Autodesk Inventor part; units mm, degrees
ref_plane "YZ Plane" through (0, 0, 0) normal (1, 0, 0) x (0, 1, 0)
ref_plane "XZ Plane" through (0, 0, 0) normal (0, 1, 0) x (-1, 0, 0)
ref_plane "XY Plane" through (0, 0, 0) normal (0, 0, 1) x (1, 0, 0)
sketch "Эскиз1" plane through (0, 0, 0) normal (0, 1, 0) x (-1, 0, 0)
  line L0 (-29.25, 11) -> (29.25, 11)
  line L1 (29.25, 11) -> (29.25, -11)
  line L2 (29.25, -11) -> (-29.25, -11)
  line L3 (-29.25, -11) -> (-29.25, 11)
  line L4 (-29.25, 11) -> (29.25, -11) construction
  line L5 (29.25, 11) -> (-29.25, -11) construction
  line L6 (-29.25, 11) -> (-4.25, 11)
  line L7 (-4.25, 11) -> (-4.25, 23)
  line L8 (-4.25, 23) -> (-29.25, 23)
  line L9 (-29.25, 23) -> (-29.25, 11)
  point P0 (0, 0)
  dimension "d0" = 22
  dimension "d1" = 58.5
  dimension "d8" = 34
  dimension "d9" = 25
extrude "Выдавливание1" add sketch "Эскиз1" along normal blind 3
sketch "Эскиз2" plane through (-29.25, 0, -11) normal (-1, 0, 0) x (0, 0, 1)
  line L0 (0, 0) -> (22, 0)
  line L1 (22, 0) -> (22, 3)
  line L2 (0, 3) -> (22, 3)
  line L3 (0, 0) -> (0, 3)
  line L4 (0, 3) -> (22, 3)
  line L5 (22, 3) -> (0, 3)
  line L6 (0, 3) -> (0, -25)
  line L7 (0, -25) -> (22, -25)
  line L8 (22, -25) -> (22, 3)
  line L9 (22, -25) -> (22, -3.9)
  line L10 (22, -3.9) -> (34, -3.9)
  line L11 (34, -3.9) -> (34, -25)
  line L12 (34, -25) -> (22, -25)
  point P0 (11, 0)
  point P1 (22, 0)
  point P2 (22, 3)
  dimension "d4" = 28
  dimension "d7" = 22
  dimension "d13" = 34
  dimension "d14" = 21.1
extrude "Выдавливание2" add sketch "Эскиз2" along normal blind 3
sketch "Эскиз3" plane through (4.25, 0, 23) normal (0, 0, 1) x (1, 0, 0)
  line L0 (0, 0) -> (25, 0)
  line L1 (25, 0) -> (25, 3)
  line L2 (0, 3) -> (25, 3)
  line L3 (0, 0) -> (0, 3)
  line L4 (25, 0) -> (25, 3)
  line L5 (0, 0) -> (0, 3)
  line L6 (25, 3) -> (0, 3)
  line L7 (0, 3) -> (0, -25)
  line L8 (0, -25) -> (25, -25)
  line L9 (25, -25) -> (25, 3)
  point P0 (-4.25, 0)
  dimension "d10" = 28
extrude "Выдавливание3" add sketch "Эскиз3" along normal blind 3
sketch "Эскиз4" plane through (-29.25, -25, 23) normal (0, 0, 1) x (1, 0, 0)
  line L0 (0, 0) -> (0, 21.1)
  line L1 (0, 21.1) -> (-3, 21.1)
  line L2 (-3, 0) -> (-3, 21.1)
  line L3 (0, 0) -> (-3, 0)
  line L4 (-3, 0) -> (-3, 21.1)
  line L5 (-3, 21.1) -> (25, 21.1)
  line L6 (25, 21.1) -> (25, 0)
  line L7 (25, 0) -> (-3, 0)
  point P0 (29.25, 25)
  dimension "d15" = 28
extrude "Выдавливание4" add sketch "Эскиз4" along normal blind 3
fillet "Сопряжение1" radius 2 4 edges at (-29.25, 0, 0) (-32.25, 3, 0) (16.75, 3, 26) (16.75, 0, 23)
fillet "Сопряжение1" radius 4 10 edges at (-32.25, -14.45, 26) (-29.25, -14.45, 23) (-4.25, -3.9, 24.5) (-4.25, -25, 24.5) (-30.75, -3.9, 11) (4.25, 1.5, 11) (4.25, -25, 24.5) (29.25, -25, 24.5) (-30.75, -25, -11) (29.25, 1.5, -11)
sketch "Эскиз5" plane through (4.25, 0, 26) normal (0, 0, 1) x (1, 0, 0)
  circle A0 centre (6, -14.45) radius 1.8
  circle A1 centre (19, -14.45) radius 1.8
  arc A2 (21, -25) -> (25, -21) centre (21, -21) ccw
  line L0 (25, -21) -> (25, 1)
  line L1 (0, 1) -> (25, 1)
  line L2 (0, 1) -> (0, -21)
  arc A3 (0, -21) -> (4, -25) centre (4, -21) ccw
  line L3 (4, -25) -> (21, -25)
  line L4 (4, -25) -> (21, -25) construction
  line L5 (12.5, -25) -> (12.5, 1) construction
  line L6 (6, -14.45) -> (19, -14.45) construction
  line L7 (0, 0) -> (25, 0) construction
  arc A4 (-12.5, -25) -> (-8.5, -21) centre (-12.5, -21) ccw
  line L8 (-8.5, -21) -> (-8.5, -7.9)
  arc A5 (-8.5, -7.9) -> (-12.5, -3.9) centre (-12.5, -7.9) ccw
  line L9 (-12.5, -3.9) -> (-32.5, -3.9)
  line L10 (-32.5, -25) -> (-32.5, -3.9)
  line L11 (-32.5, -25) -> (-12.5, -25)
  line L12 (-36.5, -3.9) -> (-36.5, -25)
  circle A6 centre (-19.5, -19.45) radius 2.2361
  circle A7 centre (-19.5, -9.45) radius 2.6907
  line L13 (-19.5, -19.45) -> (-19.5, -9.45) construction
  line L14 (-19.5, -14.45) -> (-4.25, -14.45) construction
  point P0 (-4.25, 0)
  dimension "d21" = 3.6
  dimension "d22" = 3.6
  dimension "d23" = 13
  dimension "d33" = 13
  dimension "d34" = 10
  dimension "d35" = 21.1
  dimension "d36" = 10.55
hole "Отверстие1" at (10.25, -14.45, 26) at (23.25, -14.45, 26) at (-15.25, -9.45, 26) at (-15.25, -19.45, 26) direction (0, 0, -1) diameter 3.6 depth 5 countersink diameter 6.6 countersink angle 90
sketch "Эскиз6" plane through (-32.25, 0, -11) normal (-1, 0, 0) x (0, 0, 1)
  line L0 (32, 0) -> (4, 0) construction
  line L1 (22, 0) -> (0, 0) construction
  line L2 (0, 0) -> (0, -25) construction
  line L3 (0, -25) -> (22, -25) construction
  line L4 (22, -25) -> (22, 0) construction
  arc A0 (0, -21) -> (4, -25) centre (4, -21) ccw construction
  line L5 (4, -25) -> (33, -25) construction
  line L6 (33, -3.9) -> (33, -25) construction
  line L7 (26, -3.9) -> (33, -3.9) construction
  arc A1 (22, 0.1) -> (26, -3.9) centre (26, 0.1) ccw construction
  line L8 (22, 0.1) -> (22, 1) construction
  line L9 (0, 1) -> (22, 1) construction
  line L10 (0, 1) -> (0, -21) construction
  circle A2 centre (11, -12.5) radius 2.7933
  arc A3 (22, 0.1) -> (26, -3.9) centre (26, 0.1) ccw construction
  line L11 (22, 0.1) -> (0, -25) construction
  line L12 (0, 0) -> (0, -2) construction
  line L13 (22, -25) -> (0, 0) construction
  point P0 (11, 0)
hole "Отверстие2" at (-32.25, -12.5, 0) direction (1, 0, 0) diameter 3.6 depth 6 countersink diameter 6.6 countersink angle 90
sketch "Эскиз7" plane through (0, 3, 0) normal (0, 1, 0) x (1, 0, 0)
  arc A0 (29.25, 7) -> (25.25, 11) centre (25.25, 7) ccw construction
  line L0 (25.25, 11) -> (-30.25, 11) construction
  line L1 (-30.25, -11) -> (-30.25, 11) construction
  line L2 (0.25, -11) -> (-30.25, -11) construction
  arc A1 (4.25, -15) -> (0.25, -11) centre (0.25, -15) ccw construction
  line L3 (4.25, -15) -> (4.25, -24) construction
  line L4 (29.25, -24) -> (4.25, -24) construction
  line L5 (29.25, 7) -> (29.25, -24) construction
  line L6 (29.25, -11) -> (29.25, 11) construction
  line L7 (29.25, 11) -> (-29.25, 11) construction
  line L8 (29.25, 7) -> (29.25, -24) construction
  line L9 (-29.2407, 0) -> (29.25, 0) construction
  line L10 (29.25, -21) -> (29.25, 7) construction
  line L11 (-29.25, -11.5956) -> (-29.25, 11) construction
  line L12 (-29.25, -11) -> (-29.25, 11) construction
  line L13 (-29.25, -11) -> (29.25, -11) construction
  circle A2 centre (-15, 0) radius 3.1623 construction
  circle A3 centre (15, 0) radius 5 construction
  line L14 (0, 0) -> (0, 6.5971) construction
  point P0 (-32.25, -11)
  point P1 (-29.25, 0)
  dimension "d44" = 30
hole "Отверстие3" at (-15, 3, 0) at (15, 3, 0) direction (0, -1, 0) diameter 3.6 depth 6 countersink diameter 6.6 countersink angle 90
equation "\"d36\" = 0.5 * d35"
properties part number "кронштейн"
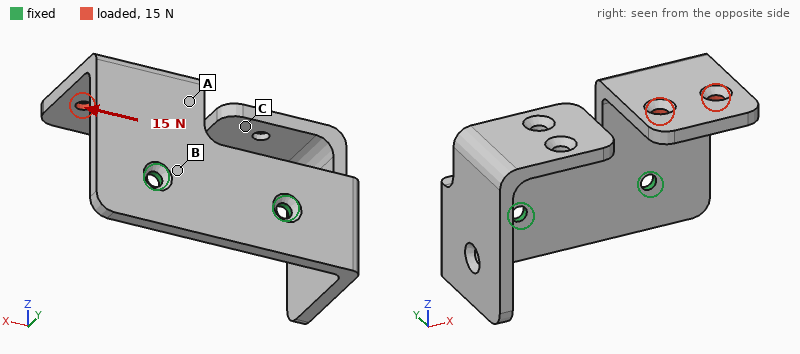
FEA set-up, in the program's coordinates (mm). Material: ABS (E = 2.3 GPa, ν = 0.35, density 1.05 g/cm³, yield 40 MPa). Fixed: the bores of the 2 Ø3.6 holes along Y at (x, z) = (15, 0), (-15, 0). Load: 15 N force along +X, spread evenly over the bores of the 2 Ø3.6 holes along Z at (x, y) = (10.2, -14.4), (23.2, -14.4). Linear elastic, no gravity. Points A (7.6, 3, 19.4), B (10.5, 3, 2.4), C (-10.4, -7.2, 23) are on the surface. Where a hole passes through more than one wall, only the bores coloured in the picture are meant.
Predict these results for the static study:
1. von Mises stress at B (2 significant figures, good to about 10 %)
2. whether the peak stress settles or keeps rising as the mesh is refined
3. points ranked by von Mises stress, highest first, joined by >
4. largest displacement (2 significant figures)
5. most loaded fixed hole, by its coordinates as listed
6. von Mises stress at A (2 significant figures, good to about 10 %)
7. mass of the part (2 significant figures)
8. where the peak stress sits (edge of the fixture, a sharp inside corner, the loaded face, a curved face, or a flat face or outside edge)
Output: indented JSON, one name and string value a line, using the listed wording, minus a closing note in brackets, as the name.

{
  "von Mises stress at B": "2.1 MPa",
  "whether the peak stress settles or keeps rising as the mesh is refined": "keeps rising",
  "points ranked by von Mises stress, highest first, joined by >": "A > B > C",
  "largest displacement": "0.76 mm",
  "most loaded fixed hole, by its coordinates as listed": "(15, 0)",
  "von Mises stress at A": "4.8 MPa",
  "mass of the part": "11 g",
  "where the peak stress sits": "edge of the fixture"
}
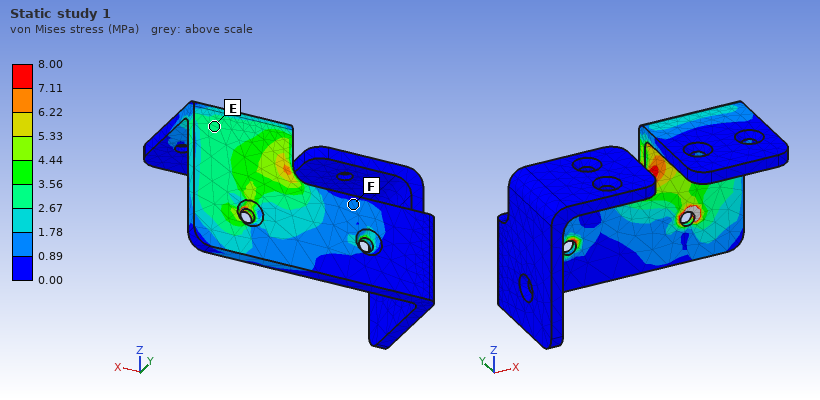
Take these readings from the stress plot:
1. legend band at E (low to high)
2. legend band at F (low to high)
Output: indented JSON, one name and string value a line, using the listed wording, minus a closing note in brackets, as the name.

{
  "legend band at E": "2.67 to 3.56 MPa",
  "legend band at F": "0.89 to 1.78 MPa"
}
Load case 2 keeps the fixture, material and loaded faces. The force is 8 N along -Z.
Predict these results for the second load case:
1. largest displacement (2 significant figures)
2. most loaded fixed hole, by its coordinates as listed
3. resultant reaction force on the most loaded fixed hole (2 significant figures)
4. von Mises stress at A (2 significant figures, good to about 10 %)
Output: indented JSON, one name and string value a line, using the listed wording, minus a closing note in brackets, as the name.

{
  "largest displacement": "0.83 mm",
  "most loaded fixed hole, by its coordinates as listed": "(15, 0)",
  "resultant reaction force on the most loaded fixed hole": "8.7 N",
  "von Mises stress at A": "3.3 MPa"
}
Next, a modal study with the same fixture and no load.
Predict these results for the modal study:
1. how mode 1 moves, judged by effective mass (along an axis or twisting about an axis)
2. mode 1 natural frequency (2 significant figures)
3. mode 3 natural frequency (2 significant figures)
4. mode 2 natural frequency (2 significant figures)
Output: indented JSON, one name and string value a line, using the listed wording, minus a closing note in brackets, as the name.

{
  "how mode 1 moves, judged by effective mass": "along X",
  "mode 1 natural frequency": "270 Hz",
  "mode 3 natural frequency": "360 Hz",
  "mode 2 natural frequency": "290 Hz"
}
